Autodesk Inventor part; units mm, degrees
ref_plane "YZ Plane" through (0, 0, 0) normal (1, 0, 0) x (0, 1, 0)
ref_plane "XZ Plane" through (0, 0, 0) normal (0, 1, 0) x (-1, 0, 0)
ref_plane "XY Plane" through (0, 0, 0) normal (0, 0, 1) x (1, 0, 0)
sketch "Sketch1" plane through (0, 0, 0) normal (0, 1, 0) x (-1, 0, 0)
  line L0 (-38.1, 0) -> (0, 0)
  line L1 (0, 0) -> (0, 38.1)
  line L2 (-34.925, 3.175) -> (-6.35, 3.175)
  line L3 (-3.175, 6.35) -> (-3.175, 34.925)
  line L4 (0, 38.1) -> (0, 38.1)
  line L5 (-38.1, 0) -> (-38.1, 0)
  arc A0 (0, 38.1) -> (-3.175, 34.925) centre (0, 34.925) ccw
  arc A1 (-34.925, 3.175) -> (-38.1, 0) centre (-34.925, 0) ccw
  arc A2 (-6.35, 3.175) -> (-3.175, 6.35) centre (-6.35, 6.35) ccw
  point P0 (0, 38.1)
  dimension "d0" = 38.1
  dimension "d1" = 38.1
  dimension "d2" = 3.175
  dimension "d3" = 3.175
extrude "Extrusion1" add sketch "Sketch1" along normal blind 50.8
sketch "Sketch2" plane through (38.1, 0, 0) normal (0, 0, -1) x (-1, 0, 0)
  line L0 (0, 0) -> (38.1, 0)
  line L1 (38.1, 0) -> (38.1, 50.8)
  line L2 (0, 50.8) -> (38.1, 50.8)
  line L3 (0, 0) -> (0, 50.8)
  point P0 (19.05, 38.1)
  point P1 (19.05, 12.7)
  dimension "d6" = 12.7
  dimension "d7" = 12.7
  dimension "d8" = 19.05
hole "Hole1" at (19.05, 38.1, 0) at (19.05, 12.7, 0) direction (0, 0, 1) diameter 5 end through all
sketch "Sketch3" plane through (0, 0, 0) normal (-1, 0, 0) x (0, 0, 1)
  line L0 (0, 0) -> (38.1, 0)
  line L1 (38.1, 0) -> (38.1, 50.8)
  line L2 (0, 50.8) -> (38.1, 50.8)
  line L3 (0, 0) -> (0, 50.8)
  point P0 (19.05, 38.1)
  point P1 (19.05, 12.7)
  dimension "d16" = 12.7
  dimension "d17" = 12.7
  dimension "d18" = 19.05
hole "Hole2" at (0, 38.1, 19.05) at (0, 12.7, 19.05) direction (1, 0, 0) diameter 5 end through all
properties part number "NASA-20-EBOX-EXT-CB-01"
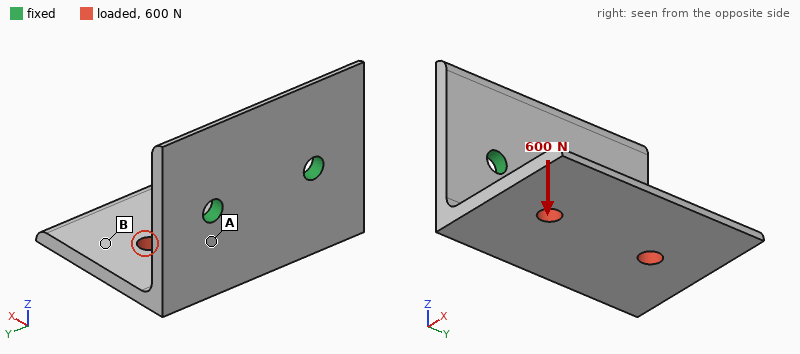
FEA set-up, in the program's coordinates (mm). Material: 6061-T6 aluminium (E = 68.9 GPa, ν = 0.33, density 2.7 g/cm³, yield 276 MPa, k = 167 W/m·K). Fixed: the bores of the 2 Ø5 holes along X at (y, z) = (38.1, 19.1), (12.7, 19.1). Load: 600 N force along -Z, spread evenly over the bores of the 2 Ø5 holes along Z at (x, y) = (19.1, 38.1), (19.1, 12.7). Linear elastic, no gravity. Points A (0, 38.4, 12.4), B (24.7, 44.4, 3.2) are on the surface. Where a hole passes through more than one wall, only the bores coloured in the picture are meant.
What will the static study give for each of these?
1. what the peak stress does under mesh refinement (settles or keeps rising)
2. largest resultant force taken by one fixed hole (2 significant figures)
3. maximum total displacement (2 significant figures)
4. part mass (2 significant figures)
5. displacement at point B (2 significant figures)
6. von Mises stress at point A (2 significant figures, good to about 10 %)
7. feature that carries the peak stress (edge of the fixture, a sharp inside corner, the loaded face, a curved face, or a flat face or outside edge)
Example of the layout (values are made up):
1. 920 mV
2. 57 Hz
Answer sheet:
1. keeps rising
2. 310 N
3. 0.81 mm
4. 31 g
5. 0.49 mm
6. 120 MPa
7. edge of the fixture
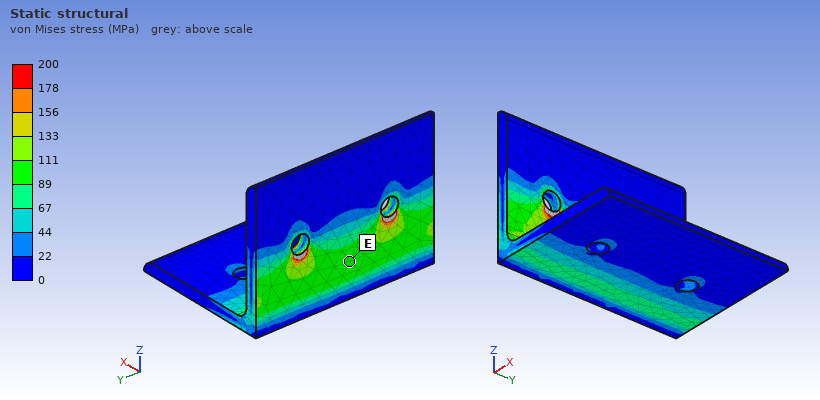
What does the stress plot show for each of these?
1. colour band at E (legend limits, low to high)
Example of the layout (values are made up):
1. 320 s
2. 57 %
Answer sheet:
1. 89 to 111 MPa
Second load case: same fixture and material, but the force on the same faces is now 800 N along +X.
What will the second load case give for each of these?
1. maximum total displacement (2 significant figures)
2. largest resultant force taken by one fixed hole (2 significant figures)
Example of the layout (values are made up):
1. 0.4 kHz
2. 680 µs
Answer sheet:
1. 0.46 mm
2. 400 N
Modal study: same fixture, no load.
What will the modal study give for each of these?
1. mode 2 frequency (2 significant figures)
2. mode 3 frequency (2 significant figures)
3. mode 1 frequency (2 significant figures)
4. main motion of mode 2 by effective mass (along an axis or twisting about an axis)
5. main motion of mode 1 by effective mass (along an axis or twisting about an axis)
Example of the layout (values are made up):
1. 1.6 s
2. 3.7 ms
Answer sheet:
1. 2400 Hz
2. 3900 Hz
3. 1200 Hz
4. along Y
5. along Z
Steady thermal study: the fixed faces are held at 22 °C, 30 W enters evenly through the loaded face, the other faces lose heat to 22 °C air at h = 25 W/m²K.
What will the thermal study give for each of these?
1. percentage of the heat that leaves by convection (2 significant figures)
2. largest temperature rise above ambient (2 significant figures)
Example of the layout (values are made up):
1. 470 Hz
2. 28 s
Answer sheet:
1. 12 %
2. 39 K
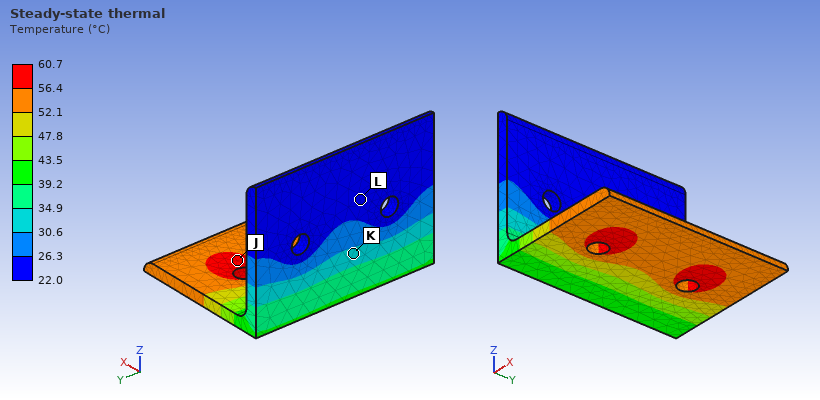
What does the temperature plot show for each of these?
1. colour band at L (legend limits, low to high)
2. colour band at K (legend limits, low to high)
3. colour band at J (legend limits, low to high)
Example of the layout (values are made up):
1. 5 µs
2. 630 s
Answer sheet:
1. 22.0 to 26.3 °C
2. 30.6 to 34.9 °C
3. 56.4 to 60.7 °C
